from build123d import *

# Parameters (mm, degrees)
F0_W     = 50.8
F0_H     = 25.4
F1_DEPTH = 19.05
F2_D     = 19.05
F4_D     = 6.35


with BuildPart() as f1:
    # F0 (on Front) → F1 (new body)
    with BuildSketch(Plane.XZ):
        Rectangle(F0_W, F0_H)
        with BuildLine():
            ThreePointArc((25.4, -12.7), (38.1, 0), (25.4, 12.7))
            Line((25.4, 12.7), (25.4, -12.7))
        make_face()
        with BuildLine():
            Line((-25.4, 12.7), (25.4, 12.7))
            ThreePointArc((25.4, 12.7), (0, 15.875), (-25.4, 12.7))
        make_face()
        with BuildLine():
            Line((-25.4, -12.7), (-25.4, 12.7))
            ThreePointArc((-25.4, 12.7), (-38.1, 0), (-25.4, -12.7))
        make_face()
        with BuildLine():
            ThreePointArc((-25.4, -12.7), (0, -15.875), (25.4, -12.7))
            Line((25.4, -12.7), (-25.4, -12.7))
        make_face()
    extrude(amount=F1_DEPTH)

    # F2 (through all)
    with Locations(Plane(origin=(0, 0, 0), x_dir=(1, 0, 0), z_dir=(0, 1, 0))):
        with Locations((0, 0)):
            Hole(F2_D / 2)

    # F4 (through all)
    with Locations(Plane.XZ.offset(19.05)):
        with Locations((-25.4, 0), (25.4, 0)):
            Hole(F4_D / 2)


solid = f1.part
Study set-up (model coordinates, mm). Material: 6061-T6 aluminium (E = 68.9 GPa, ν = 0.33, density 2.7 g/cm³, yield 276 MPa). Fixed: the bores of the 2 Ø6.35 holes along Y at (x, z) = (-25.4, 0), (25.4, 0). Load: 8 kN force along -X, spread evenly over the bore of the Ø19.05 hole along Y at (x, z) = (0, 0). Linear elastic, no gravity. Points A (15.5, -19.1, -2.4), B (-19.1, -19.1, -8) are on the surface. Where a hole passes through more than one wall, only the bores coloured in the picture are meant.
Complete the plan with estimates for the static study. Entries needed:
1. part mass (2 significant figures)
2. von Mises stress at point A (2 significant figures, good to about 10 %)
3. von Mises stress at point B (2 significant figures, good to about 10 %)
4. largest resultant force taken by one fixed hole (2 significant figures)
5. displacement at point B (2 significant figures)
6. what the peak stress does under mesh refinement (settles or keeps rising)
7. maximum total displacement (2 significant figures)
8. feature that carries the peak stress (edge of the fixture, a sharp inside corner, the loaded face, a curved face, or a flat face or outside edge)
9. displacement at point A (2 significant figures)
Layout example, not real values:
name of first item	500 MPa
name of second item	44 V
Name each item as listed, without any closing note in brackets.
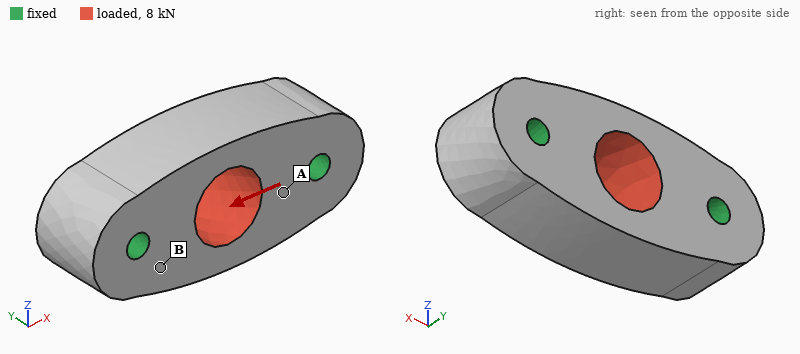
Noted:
part mass	86 g
von Mises stress at point A	11 MPa
von Mises stress at point B	6.2 MPa
largest resultant force taken by one fixed hole	4.0 kN
displacement at point B	1.6 µm
what the peak stress does under mesh refinement	keeps rising
maximum total displacement	3.7 µm
feature that carries the peak stress	edge of the fixture
displacement at point A	1.4 µm
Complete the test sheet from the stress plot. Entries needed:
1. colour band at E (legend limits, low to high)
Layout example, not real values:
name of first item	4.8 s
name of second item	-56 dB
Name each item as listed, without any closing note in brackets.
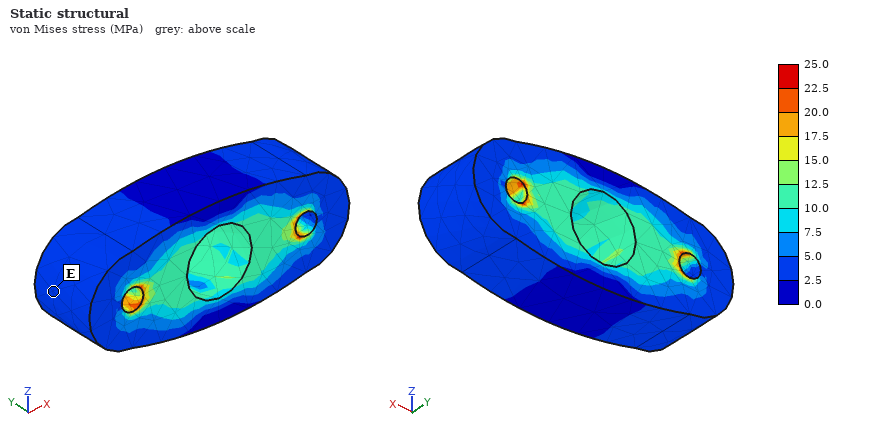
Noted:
colour band at E	2.5 to 5.0 MPa
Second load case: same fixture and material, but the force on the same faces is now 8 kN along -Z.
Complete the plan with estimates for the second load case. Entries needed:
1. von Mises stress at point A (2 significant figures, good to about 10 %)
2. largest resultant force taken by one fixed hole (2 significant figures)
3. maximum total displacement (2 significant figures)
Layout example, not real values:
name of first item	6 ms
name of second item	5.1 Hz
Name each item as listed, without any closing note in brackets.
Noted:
von Mises stress at point A	18 MPa
largest resultant force taken by one fixed hole	4.0 kN
maximum total displacement	12 µm
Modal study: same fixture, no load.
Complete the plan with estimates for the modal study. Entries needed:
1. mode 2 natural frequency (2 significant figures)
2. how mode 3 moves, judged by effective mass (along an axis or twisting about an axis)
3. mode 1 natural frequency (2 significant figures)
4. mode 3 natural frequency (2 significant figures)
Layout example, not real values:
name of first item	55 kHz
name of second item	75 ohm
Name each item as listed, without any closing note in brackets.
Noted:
mode 2 natural frequency	23 kHz
how mode 3 moves, judged by effective mass	along Z
mode 1 natural frequency	22 kHz
mode 3 natural frequency	25 kHz
